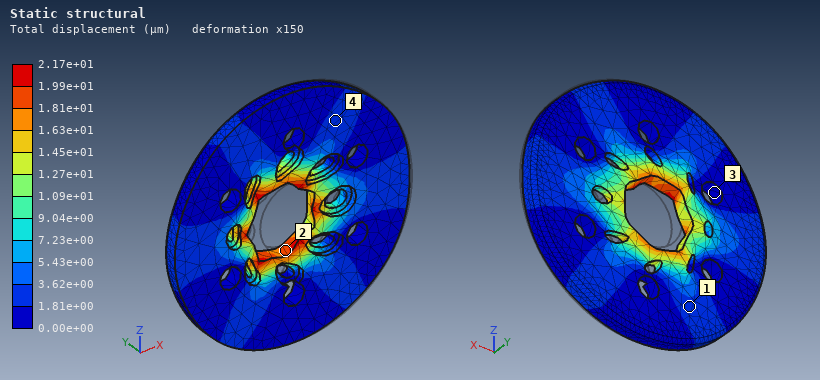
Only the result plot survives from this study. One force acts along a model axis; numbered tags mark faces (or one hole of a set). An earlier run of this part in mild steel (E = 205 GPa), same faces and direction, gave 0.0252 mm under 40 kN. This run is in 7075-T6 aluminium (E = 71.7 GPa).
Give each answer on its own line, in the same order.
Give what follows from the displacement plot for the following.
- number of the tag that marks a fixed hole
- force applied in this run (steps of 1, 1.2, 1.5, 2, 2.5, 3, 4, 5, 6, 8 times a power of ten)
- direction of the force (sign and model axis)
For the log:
3
12 kN
-X
